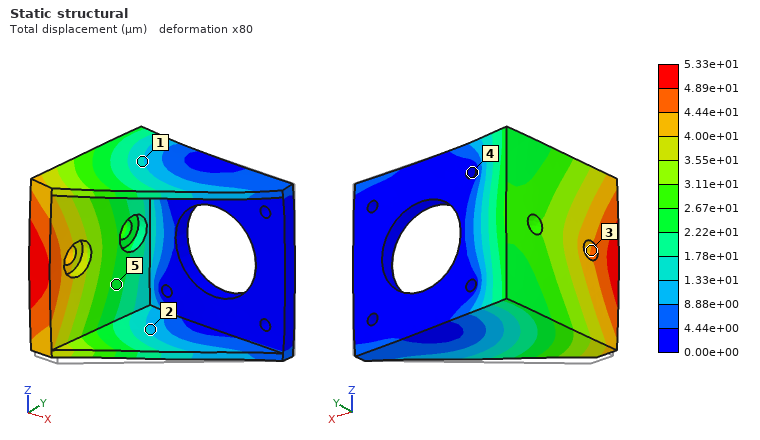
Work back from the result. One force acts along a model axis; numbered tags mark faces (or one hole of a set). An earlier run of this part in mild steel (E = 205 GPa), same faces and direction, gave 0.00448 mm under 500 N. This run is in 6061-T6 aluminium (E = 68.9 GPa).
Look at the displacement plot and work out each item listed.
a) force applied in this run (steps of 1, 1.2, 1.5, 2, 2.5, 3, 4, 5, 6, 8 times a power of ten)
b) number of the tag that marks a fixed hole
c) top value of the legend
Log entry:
2 kN
4
5.33e+01 µm
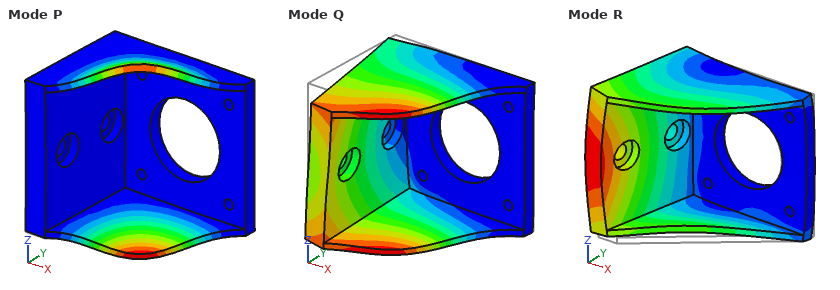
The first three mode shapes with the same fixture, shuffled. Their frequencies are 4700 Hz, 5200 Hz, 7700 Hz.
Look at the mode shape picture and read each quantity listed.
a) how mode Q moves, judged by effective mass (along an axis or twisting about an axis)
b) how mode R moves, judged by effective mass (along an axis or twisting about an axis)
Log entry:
along Z
along X
